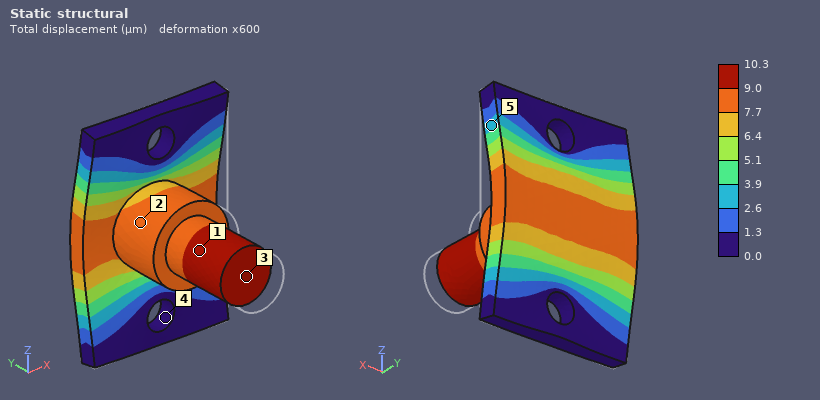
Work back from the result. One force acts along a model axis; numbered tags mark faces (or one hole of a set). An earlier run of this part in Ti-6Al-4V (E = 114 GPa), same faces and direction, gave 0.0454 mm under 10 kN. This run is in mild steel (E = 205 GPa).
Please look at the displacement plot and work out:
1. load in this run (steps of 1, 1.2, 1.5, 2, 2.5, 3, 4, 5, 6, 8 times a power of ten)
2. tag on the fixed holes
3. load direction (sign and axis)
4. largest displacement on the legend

4 kN
4
+Y
10.3 µm
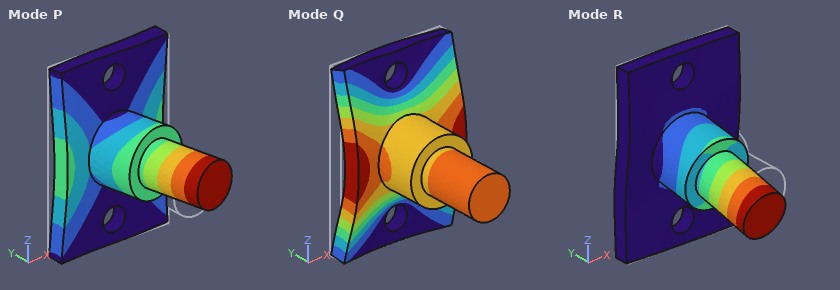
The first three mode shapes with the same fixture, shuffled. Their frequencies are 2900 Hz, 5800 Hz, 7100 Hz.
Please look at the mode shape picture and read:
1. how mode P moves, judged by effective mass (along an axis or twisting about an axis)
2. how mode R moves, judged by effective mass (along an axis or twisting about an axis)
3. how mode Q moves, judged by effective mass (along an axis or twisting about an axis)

along X
along Z
along Y
